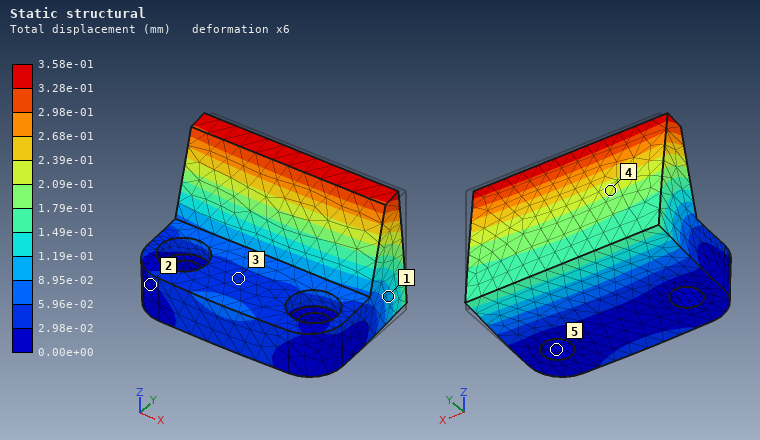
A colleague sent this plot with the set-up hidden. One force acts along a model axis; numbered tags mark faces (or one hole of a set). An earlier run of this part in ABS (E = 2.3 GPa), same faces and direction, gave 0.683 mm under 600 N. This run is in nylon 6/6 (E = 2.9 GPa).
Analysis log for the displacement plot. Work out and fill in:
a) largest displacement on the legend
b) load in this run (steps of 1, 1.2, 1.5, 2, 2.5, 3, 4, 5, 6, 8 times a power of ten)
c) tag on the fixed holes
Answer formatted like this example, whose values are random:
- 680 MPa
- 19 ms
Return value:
- 3.58e-01 mm
- 400 N
- 5
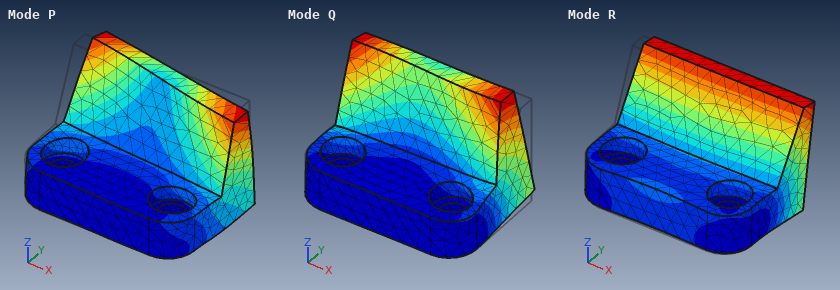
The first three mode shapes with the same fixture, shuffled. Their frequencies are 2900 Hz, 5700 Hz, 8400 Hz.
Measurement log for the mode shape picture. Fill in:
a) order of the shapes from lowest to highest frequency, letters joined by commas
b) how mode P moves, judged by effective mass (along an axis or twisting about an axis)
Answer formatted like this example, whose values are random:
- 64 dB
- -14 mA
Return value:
- R, Q, P
- along X
